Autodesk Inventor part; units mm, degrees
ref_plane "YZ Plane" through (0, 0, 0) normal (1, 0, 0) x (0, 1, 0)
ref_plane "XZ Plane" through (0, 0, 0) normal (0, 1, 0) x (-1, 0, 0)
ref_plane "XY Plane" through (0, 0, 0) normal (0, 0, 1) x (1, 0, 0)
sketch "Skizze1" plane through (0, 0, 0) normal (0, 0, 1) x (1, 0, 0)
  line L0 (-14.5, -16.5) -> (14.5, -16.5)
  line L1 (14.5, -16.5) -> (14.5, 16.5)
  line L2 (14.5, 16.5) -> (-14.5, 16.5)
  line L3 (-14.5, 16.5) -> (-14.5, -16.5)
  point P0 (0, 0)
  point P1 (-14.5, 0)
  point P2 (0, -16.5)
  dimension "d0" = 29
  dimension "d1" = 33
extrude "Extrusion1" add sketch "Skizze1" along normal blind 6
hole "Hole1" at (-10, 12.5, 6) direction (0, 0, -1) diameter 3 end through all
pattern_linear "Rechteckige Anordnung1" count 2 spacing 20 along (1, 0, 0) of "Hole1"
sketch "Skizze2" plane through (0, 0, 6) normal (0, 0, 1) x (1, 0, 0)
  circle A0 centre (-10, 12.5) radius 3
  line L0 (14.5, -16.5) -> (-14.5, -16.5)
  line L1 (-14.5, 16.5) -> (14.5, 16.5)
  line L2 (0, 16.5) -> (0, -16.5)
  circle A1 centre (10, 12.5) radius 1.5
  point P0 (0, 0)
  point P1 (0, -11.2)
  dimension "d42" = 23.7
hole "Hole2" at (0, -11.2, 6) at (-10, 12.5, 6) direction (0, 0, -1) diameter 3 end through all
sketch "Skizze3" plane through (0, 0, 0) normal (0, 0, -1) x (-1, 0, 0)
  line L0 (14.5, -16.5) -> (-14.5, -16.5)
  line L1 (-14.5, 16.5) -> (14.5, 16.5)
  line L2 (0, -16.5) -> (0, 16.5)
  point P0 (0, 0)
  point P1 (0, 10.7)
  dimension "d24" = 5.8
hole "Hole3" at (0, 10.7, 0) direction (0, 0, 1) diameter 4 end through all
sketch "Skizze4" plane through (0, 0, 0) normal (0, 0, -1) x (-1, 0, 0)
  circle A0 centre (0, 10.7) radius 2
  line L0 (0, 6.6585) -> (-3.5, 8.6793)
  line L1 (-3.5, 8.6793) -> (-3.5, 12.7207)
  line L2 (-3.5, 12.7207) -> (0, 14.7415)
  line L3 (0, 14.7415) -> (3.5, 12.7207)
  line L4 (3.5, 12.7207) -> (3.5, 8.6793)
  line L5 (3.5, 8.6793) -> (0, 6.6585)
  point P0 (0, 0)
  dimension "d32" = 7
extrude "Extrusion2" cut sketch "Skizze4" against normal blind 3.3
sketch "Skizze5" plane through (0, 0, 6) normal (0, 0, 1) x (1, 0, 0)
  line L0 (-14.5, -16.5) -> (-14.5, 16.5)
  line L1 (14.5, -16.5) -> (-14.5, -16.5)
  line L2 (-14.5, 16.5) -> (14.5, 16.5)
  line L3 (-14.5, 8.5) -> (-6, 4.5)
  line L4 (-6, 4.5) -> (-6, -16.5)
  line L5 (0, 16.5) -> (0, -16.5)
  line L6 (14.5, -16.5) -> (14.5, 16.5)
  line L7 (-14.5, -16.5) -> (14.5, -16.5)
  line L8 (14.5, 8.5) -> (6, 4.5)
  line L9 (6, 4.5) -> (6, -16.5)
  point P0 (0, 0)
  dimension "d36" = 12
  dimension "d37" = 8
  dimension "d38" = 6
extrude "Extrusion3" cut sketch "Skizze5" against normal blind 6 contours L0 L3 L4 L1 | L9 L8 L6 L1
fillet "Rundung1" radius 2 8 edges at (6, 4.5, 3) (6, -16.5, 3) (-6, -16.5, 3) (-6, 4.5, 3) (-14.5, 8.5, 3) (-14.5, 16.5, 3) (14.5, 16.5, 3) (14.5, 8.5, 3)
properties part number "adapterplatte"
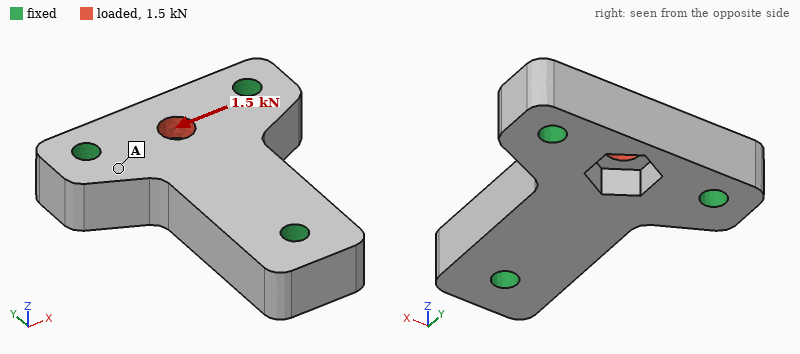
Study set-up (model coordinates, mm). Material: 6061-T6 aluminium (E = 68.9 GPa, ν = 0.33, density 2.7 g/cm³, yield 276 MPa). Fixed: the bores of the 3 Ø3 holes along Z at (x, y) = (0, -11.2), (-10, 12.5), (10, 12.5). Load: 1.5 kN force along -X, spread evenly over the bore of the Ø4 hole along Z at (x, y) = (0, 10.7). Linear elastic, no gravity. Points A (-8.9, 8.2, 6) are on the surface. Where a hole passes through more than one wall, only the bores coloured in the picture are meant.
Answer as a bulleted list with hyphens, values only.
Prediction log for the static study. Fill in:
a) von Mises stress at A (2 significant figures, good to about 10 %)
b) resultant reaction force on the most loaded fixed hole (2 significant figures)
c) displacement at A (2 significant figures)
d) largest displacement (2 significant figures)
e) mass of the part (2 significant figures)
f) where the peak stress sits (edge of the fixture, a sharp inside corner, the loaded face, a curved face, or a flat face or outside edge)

- 11 MPa
- 760 N
- 1.3 µm
- 4.1 µm
- 8.3 g
- the loaded face
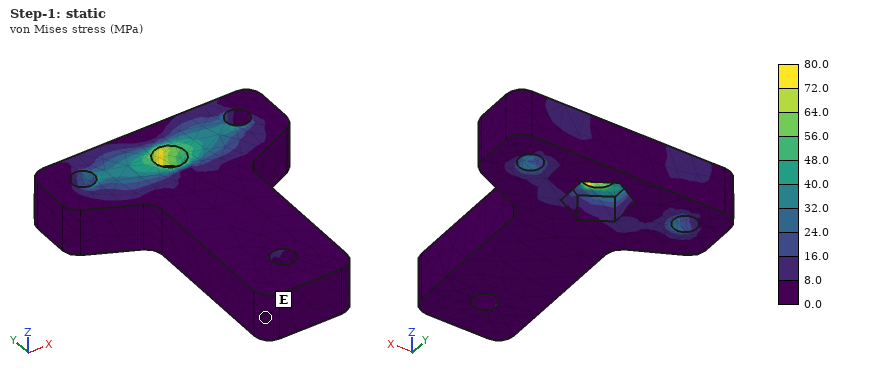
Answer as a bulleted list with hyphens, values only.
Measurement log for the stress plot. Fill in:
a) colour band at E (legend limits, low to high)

- 0.0 to 8.0 MPa
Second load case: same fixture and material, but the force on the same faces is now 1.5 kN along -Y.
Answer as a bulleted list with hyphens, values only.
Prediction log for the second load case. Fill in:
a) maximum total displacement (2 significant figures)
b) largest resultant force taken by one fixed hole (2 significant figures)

- 8.1 µm
- 540 N
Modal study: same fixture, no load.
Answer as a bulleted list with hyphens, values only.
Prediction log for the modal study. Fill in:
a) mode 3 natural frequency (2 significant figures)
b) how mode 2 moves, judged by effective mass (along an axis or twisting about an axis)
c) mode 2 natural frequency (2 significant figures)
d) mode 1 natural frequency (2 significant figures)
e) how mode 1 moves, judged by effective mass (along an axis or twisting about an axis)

- 57 kHz
- along X
- 54 kHz
- 38 kHz
- along Z
